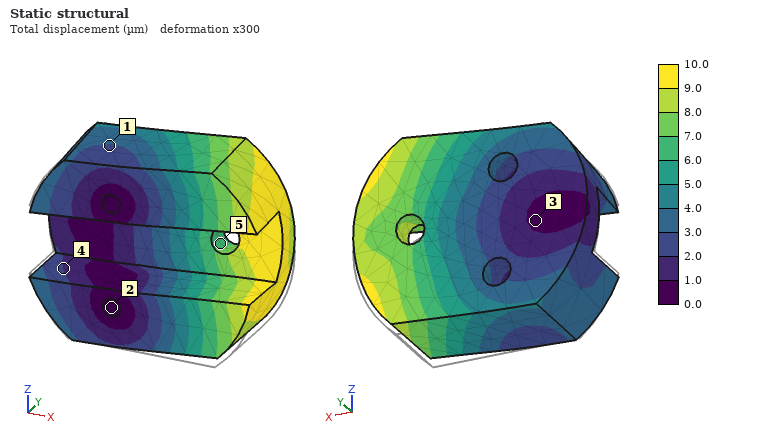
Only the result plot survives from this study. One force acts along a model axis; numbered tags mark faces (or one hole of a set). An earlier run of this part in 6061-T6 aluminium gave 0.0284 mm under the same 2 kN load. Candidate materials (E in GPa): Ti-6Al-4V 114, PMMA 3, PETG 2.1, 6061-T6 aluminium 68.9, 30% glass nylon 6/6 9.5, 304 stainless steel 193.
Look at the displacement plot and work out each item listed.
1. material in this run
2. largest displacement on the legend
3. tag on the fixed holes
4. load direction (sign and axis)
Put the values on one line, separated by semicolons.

304 stainless steel; 10.0 µm; 2; +Z
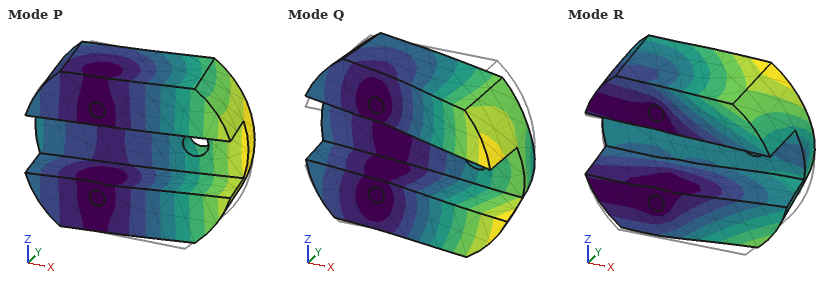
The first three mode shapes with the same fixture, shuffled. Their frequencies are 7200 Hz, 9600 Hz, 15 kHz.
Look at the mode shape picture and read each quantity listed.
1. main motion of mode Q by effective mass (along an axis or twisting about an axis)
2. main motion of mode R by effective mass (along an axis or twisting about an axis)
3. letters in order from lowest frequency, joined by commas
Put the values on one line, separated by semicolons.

along Z; along Z; P, Q, R
